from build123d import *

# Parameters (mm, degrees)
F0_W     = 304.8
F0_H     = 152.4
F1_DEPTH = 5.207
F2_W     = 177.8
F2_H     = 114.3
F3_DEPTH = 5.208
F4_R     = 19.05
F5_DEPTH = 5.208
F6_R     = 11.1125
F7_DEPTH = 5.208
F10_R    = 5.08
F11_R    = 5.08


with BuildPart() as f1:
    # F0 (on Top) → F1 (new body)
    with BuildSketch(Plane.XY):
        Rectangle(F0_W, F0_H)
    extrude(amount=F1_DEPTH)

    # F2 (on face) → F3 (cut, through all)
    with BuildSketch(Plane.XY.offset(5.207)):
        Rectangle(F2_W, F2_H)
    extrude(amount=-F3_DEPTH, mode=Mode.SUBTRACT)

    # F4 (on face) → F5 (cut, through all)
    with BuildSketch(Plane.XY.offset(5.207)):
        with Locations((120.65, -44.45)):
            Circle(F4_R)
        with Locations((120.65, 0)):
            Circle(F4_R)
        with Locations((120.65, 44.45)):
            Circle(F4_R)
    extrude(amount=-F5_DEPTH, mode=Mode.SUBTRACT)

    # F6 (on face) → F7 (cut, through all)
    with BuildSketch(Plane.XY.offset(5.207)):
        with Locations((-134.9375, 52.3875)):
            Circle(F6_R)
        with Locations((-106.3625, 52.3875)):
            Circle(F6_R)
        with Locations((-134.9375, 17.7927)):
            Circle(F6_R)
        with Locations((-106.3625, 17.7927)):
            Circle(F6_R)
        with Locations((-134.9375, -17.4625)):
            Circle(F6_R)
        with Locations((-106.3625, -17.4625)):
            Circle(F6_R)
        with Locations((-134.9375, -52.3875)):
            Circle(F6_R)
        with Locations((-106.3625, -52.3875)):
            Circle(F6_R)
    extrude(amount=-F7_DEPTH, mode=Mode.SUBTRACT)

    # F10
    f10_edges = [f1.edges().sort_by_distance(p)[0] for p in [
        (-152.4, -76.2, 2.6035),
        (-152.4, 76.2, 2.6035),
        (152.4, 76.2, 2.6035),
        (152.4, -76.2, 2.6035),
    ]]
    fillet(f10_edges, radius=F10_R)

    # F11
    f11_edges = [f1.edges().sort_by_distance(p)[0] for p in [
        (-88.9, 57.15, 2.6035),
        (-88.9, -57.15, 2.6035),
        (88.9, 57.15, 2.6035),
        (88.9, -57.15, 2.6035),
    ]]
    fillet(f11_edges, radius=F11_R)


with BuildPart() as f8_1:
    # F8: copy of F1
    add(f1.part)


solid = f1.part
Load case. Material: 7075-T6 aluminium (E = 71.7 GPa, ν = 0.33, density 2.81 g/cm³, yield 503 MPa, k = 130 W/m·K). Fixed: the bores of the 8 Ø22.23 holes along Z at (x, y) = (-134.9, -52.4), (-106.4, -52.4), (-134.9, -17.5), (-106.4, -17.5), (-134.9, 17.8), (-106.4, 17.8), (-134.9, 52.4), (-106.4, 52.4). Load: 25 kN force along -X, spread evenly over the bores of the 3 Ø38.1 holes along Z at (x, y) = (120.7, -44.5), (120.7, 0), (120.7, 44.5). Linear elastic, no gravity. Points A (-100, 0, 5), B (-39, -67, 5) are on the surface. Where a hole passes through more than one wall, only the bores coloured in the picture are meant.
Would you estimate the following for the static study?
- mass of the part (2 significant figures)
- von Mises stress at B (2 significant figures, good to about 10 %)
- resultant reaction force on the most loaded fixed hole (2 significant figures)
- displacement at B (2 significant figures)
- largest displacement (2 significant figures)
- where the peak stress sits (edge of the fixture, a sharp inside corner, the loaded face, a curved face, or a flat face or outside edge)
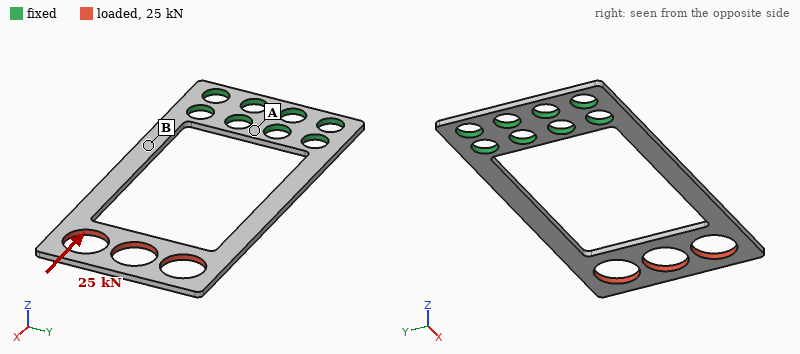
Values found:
290 g
130 MPa
11 kN
0.20 mm
0.90 mm
the loaded face
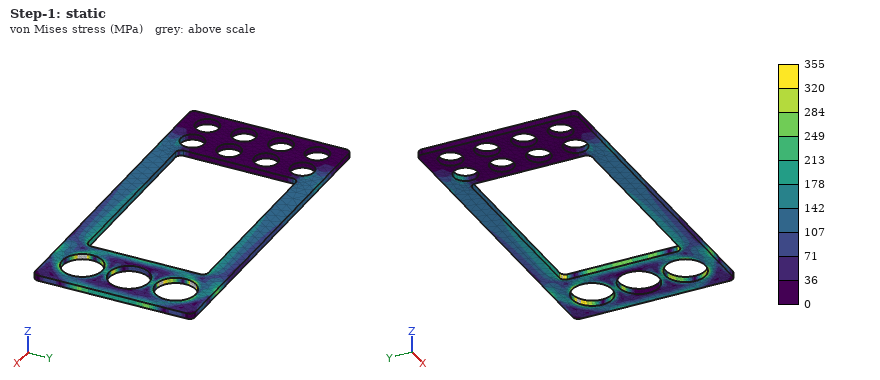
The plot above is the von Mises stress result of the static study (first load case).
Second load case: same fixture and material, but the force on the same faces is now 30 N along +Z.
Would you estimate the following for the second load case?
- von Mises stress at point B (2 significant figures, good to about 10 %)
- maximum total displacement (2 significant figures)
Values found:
28 MPa
3.9 mm
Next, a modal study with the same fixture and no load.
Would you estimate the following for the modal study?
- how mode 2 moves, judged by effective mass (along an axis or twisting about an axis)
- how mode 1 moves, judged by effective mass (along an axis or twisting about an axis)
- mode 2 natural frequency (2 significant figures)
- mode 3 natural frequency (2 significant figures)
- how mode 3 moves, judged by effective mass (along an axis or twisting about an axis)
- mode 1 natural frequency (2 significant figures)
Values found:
twisting about X
along Z
160 Hz
350 Hz
along Y
47 Hz
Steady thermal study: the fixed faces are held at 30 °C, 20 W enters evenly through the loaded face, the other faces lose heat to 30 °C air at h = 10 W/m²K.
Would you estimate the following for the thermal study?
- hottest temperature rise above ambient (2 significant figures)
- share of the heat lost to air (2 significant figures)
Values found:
71 K
70 %
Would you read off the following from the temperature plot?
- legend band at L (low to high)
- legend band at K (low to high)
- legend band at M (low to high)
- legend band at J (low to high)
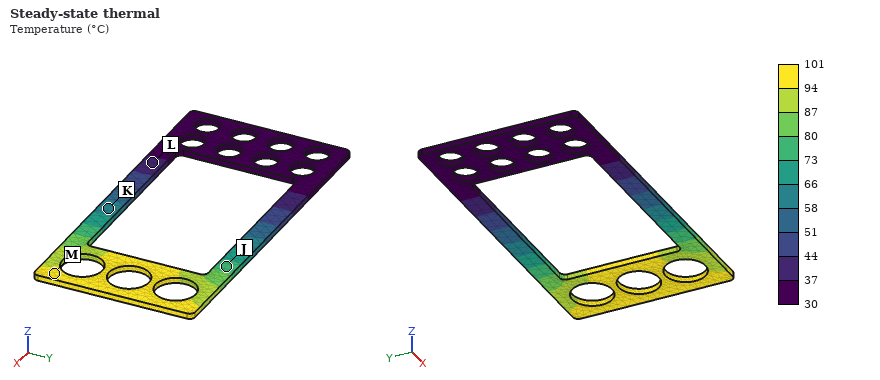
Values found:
37 to 44 °C
58 to 66 °C
94 to 101 °C
73 to 80 °C
